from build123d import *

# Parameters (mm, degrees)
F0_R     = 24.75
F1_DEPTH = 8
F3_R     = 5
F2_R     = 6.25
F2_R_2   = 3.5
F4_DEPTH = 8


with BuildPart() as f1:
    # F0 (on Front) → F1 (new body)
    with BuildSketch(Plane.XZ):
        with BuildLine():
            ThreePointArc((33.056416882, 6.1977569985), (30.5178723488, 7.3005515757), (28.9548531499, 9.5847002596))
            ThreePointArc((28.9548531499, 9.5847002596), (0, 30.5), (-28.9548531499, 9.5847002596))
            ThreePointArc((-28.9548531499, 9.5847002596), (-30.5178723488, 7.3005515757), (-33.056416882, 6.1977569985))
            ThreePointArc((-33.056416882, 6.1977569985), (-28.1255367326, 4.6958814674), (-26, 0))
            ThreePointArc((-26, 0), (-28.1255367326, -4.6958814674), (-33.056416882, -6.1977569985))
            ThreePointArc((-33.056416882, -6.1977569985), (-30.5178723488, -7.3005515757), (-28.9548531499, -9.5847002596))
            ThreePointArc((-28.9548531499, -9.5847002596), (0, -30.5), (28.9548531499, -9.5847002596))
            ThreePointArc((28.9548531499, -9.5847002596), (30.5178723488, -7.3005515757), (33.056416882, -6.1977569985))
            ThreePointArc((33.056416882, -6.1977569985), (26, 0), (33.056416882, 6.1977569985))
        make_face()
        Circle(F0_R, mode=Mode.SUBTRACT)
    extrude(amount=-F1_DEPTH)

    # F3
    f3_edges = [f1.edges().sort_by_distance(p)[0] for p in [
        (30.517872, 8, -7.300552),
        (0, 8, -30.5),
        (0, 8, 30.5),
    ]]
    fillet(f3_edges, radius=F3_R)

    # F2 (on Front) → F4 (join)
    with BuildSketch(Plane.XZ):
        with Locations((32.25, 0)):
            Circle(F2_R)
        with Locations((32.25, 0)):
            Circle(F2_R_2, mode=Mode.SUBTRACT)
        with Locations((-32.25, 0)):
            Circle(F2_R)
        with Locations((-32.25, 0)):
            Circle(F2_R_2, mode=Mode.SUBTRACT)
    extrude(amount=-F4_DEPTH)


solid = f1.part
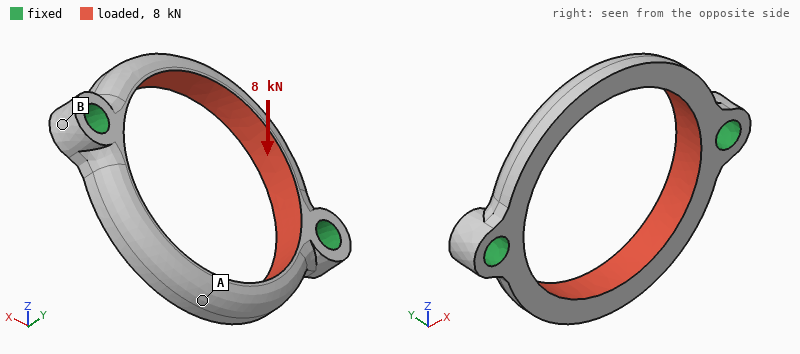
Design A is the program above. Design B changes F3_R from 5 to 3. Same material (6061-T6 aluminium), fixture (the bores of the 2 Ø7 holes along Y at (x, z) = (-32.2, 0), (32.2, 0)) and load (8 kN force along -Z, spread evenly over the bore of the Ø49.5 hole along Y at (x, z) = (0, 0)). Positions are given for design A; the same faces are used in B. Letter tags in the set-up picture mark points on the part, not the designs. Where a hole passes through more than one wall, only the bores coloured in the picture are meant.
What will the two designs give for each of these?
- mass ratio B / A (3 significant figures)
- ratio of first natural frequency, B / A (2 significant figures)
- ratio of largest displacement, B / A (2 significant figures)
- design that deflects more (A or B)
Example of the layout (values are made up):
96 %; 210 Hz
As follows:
1.07; 1.0; 0.83; A
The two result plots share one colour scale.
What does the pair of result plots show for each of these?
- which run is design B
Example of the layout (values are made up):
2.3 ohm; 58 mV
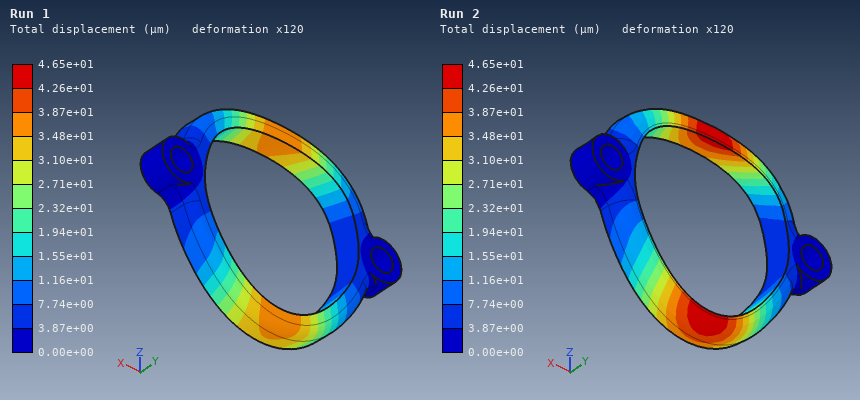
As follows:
Run 1
